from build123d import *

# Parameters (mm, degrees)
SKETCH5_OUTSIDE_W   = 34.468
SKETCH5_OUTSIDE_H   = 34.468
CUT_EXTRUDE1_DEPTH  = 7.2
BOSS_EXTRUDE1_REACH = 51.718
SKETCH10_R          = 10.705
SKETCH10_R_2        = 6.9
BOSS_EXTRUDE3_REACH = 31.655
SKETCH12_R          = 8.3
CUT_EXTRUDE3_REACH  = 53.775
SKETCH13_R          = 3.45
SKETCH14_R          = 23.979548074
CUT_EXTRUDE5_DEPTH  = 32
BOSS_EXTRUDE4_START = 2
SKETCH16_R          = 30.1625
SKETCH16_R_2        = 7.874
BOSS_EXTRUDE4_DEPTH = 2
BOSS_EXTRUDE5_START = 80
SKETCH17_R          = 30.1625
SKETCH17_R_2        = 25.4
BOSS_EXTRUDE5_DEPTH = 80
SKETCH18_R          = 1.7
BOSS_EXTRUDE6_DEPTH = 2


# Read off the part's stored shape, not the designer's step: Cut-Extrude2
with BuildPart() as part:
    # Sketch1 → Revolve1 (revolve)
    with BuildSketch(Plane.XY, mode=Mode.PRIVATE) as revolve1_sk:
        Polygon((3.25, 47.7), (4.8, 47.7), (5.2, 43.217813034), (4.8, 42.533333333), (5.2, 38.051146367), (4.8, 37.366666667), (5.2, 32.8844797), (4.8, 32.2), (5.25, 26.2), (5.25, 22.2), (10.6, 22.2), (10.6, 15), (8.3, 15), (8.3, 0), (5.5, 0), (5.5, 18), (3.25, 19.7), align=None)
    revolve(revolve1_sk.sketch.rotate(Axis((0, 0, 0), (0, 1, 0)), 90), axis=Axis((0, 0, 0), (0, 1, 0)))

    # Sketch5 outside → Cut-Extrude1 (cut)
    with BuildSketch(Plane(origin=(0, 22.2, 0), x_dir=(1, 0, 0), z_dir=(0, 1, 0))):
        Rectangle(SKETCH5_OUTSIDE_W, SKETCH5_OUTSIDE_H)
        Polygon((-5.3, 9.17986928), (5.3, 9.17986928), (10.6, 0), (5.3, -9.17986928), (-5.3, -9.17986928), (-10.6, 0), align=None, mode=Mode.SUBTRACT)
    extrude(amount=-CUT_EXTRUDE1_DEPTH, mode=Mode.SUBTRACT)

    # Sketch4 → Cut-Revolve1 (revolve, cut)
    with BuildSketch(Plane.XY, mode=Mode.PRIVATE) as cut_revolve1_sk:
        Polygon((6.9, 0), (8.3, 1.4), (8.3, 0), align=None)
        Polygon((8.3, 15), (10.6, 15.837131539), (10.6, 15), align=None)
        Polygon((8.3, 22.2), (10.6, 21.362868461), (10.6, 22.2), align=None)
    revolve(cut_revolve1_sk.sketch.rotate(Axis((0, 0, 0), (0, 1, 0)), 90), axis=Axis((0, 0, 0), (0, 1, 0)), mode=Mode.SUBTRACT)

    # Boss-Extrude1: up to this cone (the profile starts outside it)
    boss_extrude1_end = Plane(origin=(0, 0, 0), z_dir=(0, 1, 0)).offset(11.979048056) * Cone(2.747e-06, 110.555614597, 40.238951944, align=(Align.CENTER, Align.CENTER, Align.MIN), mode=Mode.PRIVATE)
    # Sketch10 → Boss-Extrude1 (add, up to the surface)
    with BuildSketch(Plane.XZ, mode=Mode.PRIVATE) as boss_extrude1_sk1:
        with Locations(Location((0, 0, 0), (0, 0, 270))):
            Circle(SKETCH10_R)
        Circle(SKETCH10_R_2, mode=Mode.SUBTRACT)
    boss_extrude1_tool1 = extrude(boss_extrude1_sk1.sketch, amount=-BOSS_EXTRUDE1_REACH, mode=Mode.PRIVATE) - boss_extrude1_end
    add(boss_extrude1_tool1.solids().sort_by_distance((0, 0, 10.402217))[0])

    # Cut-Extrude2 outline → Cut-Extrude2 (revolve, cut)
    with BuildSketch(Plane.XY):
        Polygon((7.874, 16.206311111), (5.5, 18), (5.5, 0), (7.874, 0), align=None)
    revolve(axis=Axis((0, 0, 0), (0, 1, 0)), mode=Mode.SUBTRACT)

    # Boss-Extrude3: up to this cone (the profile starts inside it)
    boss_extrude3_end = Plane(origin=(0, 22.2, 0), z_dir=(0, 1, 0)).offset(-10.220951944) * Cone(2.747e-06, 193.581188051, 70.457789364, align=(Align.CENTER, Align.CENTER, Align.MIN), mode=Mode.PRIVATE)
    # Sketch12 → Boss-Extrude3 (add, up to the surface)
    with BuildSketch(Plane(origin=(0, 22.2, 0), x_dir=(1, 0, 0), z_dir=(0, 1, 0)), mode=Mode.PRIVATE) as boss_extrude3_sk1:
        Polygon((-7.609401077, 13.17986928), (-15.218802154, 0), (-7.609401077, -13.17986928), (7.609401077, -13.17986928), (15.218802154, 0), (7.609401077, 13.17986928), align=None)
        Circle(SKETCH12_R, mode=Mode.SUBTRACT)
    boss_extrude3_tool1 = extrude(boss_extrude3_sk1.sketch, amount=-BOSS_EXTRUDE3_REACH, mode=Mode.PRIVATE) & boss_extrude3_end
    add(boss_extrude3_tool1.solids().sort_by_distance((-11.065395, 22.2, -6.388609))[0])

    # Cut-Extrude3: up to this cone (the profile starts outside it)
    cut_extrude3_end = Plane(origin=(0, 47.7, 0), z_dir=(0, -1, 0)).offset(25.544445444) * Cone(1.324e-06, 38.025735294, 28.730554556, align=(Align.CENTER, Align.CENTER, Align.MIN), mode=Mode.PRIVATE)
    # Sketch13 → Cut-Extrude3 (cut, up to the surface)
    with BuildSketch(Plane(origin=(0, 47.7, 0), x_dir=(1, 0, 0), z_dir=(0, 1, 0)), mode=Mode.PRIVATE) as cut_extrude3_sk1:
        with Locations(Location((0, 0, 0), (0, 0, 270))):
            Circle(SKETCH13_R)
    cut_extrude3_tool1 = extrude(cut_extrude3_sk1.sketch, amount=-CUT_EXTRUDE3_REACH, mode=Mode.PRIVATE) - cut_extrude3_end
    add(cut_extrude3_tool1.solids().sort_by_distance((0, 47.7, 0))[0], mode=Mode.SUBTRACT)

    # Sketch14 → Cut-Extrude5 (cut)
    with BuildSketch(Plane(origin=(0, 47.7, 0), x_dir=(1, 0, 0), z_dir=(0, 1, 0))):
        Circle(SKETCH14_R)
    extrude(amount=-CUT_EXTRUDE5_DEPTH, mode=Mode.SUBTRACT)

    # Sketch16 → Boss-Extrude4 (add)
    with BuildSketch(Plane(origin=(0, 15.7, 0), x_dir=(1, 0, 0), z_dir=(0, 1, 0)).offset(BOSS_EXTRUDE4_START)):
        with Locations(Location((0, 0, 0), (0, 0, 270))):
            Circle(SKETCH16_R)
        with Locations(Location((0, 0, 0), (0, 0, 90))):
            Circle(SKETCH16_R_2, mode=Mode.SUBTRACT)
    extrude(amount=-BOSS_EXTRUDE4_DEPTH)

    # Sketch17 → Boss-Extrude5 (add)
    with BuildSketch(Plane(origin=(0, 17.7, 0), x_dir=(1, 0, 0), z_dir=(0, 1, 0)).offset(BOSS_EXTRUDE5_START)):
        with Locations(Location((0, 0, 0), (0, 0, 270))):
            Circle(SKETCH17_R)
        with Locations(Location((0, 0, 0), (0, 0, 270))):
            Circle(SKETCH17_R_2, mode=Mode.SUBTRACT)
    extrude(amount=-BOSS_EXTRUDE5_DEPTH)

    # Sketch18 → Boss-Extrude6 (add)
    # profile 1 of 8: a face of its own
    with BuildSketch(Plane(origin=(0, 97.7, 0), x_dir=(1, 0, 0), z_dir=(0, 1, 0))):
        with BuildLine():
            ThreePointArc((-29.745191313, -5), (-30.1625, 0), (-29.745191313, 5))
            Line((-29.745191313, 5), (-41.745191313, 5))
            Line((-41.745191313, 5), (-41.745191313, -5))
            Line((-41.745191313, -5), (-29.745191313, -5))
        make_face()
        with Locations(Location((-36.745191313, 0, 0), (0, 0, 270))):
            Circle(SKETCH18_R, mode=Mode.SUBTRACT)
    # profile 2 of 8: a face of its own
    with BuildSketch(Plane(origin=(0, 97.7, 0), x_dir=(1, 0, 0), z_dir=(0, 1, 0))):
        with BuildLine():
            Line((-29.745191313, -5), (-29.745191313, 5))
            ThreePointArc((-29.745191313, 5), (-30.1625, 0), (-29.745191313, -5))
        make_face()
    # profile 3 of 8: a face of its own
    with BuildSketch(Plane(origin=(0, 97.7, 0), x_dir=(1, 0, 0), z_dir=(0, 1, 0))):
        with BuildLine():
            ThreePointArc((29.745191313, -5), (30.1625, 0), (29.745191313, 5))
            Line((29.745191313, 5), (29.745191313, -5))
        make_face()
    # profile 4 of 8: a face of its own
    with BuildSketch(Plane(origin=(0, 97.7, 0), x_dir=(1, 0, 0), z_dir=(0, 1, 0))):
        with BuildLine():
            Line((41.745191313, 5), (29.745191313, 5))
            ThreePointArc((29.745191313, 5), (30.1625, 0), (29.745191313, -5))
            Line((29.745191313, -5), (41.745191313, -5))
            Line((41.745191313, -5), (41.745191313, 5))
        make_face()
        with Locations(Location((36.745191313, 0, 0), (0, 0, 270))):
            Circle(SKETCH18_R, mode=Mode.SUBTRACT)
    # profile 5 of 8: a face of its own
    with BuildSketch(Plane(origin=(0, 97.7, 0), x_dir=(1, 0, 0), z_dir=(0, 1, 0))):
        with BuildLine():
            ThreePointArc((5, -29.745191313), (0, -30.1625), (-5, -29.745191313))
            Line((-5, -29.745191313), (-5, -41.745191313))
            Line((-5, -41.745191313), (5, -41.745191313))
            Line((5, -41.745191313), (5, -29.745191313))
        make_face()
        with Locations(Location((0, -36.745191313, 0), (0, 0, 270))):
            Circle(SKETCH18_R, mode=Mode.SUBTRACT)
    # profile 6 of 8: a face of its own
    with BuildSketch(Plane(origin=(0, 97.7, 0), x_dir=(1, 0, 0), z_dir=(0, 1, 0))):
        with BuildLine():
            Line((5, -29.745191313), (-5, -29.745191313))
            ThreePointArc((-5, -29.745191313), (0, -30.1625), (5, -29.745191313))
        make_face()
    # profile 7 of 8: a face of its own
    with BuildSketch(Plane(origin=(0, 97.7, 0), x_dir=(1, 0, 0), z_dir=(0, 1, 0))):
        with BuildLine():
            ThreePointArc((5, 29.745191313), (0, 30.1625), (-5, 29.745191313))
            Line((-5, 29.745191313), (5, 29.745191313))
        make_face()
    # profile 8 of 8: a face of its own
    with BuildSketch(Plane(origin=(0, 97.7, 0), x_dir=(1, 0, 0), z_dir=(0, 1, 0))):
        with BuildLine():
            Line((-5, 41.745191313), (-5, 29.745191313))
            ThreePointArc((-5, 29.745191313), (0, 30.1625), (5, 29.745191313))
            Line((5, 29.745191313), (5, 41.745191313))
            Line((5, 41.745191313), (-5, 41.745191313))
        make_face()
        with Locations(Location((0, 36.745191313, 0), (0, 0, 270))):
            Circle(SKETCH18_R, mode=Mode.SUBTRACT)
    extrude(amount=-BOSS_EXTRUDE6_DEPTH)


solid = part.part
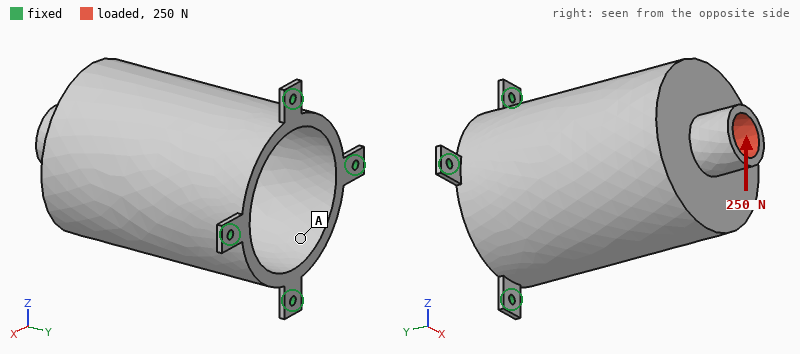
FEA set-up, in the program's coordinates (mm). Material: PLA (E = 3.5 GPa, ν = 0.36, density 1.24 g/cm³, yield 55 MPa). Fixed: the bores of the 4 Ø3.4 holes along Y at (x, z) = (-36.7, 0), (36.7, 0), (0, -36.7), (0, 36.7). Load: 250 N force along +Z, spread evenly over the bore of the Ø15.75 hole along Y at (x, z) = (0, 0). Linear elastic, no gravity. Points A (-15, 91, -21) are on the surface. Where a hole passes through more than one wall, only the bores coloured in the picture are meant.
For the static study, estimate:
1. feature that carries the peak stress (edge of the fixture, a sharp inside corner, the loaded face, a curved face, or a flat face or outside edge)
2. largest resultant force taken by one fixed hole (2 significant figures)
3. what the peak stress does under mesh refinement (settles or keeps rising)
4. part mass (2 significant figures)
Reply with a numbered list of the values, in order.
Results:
1. edge of the fixture
2. 360 N
3. keeps rising
4. 93 g
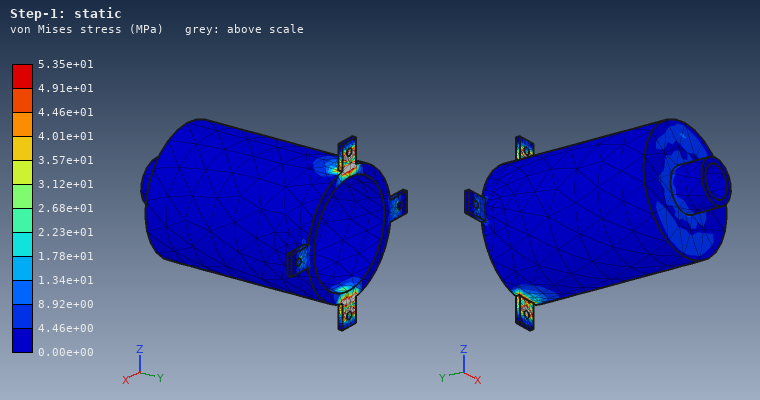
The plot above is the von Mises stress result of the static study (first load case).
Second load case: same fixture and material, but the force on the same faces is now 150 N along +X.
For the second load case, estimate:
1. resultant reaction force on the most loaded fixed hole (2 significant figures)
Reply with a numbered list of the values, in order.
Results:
1. 220 N
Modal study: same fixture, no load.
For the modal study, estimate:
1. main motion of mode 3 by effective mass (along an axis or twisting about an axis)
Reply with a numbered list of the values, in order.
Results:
1. along Y
